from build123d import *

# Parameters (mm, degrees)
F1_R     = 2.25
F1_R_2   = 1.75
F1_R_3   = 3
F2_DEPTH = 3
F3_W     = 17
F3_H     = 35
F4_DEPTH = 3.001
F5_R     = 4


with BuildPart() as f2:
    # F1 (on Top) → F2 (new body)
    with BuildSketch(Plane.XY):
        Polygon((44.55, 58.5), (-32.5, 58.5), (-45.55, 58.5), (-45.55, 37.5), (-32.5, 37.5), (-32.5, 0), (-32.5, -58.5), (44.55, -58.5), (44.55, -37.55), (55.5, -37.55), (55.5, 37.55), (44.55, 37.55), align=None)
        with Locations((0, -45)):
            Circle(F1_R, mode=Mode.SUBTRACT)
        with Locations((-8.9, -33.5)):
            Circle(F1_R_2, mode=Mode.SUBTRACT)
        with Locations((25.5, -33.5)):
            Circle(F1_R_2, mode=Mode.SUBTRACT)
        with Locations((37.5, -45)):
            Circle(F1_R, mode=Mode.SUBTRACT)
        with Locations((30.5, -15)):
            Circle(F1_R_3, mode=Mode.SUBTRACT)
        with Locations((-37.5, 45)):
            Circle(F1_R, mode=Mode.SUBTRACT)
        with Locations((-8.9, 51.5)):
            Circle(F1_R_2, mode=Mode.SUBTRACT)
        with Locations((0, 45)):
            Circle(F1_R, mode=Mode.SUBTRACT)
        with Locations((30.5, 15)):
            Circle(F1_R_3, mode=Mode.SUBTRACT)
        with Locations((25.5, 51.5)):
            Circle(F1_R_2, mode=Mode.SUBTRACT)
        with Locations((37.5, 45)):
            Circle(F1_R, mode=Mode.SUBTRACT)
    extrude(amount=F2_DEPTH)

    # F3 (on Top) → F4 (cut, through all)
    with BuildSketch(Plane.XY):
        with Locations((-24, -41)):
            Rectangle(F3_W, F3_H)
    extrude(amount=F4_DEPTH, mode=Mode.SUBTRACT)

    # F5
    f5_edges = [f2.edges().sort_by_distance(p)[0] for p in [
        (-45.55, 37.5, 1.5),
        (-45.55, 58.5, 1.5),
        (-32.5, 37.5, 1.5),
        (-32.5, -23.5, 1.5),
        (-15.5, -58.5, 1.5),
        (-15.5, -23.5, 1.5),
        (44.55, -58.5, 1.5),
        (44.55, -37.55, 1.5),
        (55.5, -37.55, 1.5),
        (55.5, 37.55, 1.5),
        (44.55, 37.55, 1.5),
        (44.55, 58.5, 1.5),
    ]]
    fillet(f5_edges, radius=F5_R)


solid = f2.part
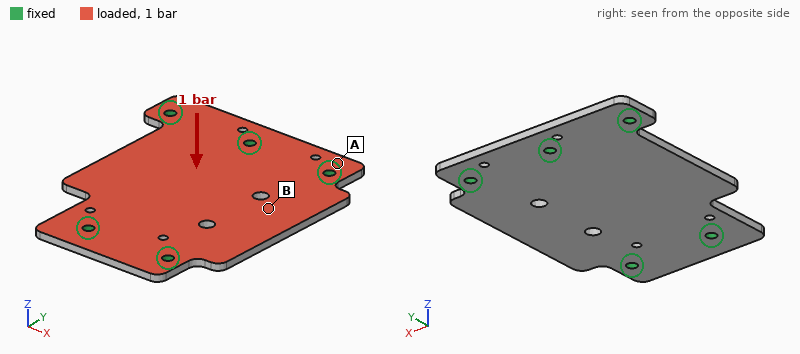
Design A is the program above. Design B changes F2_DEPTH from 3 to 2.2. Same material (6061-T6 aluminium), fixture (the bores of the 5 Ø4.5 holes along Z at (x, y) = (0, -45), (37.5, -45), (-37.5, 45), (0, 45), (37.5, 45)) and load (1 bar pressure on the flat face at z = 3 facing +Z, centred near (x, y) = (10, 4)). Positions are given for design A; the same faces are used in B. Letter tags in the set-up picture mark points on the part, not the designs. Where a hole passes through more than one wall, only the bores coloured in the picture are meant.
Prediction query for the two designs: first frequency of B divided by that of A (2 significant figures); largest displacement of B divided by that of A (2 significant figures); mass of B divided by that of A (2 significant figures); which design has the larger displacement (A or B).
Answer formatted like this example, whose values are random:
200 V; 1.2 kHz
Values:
0.75; 2.5; 0.73; B
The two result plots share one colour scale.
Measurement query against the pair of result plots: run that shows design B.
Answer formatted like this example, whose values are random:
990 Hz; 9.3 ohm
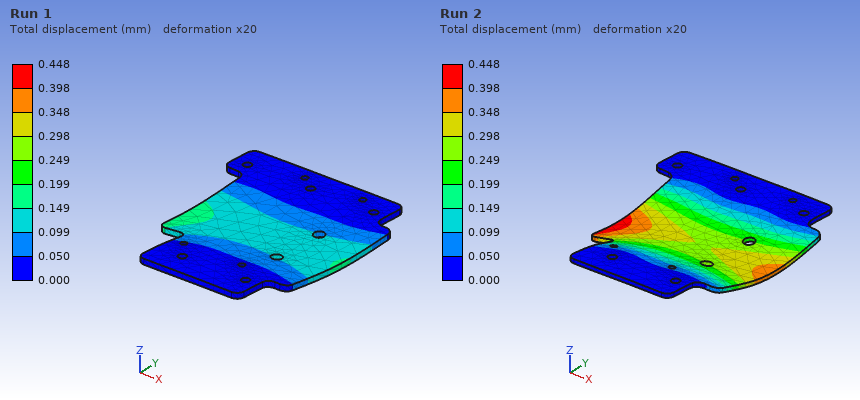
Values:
Run 2
